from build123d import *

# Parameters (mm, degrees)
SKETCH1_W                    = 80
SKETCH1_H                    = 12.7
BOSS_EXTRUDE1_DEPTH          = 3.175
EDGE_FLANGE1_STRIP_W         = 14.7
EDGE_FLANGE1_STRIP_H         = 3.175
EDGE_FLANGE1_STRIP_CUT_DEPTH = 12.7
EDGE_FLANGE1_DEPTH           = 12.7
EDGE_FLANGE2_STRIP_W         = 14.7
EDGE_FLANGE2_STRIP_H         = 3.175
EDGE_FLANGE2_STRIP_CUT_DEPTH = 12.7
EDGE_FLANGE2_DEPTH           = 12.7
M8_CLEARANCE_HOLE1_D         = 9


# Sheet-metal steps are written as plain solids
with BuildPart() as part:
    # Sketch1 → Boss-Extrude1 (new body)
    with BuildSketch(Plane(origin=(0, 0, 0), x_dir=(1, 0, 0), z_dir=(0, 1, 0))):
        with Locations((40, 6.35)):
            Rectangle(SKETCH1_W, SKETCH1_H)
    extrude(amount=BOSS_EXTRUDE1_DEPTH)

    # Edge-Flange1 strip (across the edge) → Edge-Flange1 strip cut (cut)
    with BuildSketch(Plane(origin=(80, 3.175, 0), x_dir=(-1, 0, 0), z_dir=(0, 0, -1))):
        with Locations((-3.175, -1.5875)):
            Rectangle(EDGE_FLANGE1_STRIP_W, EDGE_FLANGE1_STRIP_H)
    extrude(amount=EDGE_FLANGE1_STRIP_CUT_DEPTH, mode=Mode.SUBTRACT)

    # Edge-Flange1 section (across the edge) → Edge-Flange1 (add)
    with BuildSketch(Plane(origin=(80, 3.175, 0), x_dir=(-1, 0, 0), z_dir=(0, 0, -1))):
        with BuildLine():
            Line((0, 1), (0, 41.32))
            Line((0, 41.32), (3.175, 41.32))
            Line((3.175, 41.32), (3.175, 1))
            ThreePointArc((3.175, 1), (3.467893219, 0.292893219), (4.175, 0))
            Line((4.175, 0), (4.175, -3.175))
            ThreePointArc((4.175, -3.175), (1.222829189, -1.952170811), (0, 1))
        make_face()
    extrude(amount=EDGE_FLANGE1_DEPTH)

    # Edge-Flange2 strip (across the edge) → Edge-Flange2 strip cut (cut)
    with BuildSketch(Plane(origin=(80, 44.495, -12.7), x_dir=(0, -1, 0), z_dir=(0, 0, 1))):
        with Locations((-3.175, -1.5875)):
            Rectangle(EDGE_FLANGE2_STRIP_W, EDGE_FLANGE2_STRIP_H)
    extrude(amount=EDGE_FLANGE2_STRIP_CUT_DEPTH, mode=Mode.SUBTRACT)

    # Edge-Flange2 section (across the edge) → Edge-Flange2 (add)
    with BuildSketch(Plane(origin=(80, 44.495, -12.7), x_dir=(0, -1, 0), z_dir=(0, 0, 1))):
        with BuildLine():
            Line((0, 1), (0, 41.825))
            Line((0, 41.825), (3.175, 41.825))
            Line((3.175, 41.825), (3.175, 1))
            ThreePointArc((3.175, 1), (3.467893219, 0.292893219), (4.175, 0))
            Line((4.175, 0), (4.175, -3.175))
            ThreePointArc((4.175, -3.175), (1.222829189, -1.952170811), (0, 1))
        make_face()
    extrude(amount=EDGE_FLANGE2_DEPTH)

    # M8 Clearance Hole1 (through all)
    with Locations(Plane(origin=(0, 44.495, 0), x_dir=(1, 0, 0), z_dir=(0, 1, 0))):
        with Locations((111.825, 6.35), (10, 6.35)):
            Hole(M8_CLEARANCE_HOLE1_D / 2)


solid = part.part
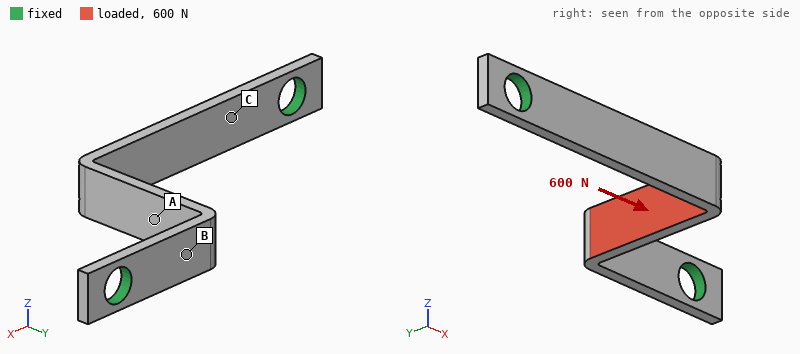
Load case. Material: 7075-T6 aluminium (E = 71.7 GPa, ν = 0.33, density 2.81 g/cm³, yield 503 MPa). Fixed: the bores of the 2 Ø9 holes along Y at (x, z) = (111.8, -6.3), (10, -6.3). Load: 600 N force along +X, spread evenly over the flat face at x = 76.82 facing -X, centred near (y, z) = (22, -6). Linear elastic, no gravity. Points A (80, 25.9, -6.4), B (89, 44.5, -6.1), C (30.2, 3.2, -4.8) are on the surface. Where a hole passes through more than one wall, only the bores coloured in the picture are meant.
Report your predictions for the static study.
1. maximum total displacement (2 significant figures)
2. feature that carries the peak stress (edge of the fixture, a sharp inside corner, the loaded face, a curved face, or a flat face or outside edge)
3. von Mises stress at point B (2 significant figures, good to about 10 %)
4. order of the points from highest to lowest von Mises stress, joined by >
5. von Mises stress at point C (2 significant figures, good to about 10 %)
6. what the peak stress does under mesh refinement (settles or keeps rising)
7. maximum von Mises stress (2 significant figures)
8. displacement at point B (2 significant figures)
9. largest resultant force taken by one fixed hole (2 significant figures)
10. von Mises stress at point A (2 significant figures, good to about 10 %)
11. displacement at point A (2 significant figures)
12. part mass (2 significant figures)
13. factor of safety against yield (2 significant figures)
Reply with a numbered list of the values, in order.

1. 0.28 mm
2. a flat face or outside edge
3. 38 MPa
4. A > B > C
5. 14 MPa
6. settles
7. 120 MPa
8. 0.091 mm
9. 310 N
10. 110 MPa
11. 0.26 mm
12. 17 g
13. 4.1
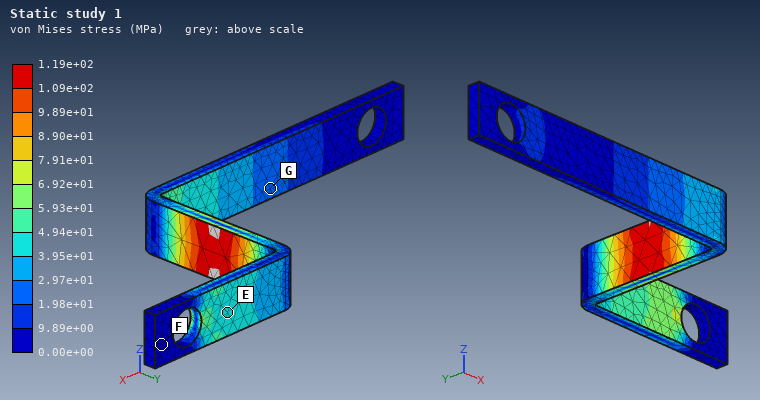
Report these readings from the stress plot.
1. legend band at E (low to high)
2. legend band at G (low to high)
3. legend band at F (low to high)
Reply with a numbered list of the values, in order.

1. 3.95e+01 to 4.94e+01 MPa
2. 1.98e+01 to 2.97e+01 MPa
3. 0.00e+00 to 9.89e+00 MPa
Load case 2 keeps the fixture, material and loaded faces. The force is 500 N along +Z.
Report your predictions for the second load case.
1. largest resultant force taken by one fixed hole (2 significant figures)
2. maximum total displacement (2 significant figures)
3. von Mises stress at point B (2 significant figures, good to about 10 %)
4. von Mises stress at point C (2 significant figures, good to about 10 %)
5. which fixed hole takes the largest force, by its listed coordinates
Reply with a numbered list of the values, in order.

1. 290 N
2. 0.48 mm
3. 36 MPa
4. 26 MPa
5. (111.8, -6.3)
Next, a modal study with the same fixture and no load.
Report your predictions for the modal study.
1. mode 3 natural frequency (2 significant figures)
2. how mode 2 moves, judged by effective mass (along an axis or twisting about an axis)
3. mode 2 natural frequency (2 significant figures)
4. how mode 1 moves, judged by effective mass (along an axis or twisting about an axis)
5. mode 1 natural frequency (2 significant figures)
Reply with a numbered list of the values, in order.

1. 3400 Hz
2. along Z
3. 1900 Hz
4. along Y
5. 1400 Hz
